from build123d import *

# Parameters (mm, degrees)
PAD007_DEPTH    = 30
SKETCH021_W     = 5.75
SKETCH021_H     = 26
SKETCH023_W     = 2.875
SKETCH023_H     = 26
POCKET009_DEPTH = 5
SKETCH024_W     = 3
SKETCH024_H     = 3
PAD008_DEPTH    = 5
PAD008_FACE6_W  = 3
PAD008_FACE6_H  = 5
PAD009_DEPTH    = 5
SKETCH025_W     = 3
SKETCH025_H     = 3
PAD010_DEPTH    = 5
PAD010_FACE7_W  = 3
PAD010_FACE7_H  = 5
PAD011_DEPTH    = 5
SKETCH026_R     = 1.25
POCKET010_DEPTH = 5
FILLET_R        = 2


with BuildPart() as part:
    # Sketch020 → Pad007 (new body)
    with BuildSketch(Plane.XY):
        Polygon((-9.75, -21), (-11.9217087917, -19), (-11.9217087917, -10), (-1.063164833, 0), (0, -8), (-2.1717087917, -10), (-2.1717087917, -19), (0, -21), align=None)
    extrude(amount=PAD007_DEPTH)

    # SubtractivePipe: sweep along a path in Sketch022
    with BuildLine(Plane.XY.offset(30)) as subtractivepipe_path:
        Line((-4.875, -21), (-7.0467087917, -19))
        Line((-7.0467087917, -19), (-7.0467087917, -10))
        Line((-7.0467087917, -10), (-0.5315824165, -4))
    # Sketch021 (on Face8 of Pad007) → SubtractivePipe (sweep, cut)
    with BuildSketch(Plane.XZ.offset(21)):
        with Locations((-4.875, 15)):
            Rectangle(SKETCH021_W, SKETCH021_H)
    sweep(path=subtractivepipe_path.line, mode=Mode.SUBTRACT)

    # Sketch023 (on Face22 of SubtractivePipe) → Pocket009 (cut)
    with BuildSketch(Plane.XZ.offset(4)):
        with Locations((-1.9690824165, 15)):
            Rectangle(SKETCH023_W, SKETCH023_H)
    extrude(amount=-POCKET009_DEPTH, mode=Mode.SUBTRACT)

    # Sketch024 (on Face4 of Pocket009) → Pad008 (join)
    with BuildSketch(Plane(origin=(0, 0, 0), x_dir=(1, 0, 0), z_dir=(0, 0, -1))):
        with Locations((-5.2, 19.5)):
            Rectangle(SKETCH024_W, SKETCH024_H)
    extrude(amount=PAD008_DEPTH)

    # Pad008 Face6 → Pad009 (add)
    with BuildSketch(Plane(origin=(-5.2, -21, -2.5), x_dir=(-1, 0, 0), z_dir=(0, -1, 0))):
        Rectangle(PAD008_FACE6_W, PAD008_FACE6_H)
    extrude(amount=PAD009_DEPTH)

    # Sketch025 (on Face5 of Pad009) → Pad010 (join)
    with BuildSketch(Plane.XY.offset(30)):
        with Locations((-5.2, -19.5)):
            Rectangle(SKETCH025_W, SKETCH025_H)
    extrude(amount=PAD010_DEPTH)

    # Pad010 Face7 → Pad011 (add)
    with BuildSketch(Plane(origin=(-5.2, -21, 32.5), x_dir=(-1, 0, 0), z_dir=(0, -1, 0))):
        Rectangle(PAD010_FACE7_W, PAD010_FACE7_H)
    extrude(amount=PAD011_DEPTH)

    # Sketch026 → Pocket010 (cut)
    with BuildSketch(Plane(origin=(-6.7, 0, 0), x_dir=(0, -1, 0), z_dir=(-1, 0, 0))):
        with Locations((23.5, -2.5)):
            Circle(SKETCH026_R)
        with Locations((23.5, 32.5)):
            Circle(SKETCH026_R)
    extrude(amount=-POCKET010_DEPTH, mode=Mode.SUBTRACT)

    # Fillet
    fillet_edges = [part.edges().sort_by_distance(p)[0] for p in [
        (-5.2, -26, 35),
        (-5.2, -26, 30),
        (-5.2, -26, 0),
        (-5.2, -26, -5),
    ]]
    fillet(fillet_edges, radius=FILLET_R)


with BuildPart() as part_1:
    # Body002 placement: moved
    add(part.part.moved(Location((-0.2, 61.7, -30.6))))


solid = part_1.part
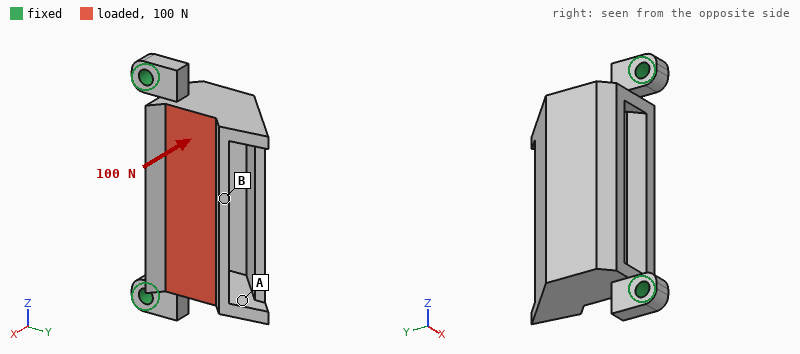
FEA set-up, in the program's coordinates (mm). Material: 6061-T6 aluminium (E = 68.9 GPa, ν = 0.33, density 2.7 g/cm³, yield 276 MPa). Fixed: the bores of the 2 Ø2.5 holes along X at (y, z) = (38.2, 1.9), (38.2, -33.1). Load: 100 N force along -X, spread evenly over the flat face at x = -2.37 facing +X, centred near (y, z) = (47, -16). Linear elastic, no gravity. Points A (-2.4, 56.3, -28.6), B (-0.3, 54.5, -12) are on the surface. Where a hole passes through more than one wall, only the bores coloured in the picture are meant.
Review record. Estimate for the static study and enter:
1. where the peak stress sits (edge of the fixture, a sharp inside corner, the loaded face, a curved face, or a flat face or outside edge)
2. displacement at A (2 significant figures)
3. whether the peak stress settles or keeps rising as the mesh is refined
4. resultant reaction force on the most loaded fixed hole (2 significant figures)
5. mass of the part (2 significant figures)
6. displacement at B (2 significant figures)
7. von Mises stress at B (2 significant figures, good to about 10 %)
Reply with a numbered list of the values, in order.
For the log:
1. edge of the fixture
2. 43 µm
3. keeps rising
4. 51 N
5. 6.8 g
6. 45 µm
7. 12 MPa
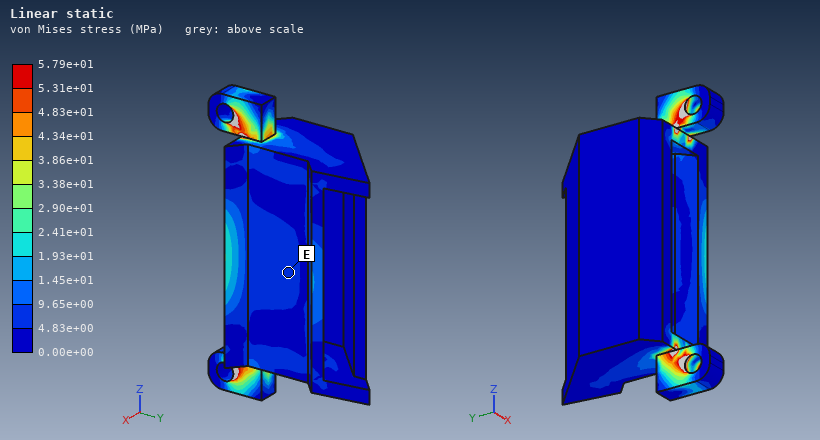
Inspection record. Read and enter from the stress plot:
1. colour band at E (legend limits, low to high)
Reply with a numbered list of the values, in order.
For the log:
1. 4.83e+00 to 9.65e+00 MPa
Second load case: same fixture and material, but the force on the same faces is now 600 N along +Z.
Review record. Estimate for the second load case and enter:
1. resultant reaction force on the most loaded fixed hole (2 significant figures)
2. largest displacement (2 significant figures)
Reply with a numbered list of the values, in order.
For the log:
1. 320 N
2. 21 µm
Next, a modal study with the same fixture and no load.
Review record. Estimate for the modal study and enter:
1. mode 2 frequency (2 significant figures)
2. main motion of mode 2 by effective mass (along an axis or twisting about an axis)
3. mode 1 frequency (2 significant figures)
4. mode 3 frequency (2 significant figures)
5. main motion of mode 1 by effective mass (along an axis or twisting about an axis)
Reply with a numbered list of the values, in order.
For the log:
1. 9300 Hz
2. twisting about Y
3. 3000 Hz
4. 13 kHz
5. along X
